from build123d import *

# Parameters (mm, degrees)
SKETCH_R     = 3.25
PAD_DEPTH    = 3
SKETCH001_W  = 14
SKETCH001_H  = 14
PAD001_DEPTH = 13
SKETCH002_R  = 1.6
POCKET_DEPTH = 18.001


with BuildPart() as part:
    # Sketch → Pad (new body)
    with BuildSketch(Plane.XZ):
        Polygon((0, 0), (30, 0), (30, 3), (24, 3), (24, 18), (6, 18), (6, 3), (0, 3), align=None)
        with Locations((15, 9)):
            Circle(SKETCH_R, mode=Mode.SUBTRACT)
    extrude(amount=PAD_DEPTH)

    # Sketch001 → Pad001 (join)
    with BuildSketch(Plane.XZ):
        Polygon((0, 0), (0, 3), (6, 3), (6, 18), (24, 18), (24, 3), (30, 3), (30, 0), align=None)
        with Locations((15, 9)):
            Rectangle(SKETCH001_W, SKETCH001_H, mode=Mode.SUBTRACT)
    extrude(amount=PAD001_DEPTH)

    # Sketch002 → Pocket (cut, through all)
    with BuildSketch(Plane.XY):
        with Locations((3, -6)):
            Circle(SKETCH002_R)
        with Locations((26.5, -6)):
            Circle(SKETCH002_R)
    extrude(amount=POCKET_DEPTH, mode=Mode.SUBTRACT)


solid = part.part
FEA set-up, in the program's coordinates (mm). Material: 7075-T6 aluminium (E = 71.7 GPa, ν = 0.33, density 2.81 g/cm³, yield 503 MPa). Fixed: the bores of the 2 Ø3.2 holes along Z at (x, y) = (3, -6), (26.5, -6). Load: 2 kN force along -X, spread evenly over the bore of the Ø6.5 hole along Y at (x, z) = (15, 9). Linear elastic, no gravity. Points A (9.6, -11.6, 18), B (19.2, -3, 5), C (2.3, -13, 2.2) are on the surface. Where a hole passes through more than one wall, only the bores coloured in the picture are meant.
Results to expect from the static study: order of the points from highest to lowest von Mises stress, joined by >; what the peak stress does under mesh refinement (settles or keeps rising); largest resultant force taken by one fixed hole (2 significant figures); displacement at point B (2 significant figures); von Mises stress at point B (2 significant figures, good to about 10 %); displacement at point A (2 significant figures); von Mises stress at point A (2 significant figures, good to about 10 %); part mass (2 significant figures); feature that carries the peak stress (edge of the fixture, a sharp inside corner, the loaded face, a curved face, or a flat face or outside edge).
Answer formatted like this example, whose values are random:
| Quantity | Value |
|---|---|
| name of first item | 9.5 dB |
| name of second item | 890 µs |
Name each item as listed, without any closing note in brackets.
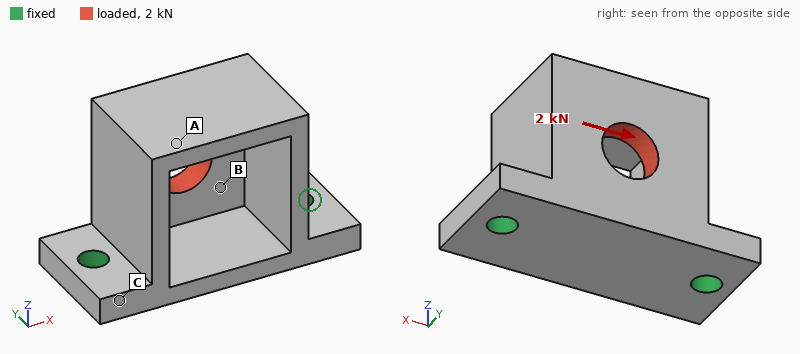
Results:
| Quantity | Value |
|---|---|
| order of the points from highest to lowest von Mises stress, joined by > | B > A > C |
| what the peak stress does under mesh refinement | keeps rising |
| largest resultant force taken by one fixed hole | 1.3 kN |
| displacement at point B | 13 µm |
| von Mises stress at point B | 62 MPa |
| displacement at point A | 54 µm |
| von Mises stress at point A | 35 MPa |
| part mass | 7.2 g |
| feature that carries the peak stress | edge of the fixture |
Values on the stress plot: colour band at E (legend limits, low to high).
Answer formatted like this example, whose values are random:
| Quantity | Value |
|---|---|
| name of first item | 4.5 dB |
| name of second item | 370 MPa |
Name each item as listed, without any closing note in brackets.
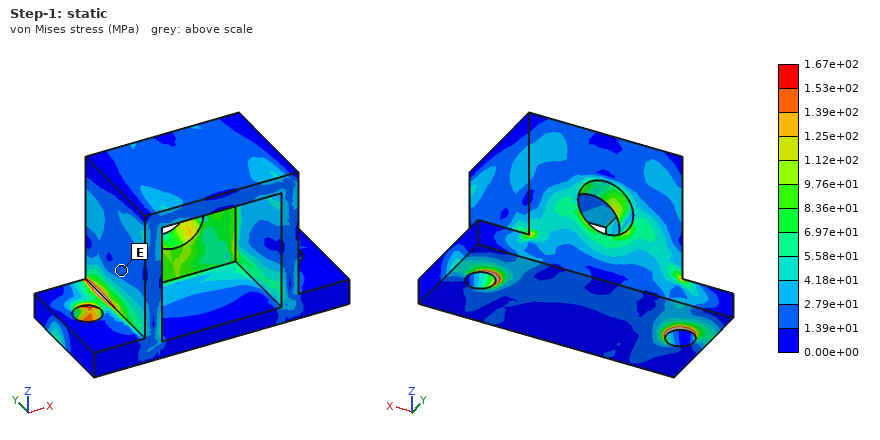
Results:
| Quantity | Value |
|---|---|
| colour band at E | 1.39e+01 to 2.79e+01 MPa |
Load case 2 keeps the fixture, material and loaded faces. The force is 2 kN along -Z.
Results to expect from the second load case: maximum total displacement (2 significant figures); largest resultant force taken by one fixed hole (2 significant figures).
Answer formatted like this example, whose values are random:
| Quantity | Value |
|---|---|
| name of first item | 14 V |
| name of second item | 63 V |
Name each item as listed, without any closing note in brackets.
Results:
| Quantity | Value |
|---|---|
| maximum total displacement | 93 µm |
| largest resultant force taken by one fixed hole | 1.1 kN |
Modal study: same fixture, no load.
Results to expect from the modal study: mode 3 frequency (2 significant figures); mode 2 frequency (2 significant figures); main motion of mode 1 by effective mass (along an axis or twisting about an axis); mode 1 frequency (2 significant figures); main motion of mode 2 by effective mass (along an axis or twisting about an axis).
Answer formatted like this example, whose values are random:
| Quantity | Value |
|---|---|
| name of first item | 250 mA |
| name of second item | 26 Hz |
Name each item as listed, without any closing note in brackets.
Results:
| Quantity | Value |
|---|---|
| mode 3 frequency | 23 kHz |
| mode 2 frequency | 10 kHz |
| main motion of mode 1 by effective mass | along Y |
| mode 1 frequency | 8000 Hz |
| main motion of mode 2 by effective mass | along X |
